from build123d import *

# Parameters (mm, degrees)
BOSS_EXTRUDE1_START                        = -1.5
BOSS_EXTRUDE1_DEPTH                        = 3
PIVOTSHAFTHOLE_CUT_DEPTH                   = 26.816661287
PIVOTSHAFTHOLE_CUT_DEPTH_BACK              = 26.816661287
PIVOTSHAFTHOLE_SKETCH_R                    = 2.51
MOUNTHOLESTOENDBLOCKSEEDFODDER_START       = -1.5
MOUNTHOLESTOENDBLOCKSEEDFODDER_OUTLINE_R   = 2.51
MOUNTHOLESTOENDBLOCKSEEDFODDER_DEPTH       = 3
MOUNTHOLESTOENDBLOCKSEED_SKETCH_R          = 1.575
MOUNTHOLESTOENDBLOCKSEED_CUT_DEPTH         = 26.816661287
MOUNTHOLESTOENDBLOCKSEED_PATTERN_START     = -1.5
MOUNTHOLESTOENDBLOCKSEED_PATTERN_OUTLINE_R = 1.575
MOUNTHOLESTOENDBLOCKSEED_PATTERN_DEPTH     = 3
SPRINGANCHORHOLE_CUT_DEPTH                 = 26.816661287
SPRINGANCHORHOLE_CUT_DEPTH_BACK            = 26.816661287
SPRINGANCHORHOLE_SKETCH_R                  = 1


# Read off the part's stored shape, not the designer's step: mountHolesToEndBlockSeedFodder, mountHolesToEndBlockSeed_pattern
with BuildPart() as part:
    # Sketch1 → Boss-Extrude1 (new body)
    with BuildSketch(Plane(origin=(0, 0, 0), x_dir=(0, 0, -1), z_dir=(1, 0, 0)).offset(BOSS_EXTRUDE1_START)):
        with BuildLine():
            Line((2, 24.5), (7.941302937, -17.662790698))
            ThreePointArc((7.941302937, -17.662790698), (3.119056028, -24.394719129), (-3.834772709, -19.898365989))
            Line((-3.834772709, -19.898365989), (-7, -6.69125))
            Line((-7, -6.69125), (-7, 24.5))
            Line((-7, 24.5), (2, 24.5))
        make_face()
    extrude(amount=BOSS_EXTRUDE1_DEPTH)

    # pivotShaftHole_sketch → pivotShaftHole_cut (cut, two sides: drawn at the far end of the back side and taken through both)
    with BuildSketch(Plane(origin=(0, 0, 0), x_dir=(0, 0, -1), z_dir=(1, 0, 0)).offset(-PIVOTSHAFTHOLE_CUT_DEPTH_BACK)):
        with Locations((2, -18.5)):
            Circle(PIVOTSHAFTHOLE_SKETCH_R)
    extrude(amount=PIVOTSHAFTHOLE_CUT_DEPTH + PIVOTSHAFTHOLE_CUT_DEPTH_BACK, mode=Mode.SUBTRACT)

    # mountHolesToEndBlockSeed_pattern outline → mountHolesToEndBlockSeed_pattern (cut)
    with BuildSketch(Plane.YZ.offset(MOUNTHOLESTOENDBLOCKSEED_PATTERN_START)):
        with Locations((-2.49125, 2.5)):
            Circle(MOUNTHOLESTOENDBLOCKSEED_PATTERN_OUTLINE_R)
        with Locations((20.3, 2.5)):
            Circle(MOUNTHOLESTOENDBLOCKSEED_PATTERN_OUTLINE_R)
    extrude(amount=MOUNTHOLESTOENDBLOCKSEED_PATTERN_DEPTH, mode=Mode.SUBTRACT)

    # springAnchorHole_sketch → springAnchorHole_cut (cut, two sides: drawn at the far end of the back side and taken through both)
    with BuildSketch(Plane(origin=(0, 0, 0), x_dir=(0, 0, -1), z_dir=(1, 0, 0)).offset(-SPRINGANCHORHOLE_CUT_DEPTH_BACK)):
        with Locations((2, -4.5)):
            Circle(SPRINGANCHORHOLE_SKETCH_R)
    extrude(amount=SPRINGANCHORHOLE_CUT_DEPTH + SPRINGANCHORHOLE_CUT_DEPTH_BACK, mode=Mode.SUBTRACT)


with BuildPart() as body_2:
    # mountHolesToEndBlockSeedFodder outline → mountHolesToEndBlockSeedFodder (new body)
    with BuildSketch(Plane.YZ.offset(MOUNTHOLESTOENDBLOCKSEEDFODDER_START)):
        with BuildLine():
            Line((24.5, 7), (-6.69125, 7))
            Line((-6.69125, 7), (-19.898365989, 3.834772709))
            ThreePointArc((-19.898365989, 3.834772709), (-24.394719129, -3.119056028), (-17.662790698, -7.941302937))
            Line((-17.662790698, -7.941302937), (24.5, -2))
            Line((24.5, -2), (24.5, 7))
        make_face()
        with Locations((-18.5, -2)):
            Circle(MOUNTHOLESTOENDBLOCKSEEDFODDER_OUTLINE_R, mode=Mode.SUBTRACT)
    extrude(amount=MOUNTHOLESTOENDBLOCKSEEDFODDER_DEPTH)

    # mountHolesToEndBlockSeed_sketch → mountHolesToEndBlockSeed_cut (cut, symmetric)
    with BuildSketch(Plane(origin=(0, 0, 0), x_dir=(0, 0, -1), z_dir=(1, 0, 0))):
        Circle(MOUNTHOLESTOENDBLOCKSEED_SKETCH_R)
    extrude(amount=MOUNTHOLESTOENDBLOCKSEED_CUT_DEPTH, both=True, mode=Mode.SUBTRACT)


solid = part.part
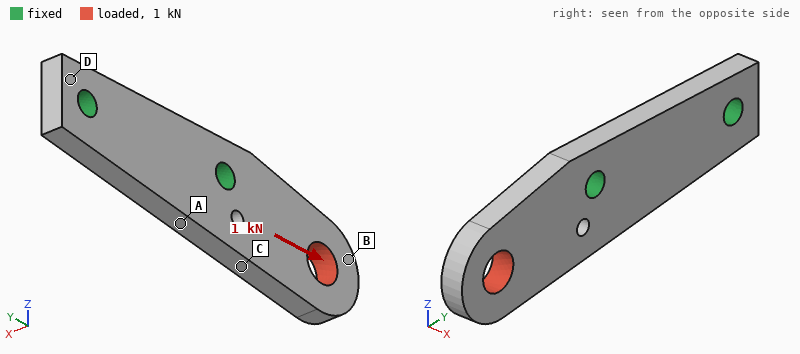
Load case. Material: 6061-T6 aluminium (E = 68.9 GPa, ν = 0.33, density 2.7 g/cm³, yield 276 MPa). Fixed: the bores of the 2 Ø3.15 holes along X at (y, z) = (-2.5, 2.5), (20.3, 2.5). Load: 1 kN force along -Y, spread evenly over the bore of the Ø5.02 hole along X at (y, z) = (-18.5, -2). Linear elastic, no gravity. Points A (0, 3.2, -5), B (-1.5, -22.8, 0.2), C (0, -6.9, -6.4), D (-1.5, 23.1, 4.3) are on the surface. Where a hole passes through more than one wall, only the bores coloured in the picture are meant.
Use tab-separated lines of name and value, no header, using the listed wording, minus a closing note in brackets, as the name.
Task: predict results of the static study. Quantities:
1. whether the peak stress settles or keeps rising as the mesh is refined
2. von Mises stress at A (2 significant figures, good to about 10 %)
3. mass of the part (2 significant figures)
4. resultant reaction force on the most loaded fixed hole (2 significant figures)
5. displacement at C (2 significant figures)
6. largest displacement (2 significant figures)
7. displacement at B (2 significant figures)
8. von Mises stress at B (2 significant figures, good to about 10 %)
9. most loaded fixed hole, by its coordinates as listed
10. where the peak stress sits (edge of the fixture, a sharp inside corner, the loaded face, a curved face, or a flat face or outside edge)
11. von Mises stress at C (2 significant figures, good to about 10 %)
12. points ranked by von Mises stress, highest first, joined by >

whether the peak stress settles or keeps rising as the mesh is refined	keeps rising
von Mises stress at A	39 MPa
mass of the part	4.2 g
resultant reaction force on the most loaded fixed hole	820 N
displacement at C	14 µm
largest displacement	35 µm
displacement at B	31 µm
von Mises stress at B	21 MPa
most loaded fixed hole, by its coordinates as listed	(-2.5, 2.5)
where the peak stress sits	edge of the fixture
von Mises stress at C	54 MPa
points ranked by von Mises stress, highest first, joined by >	C > A > B > D
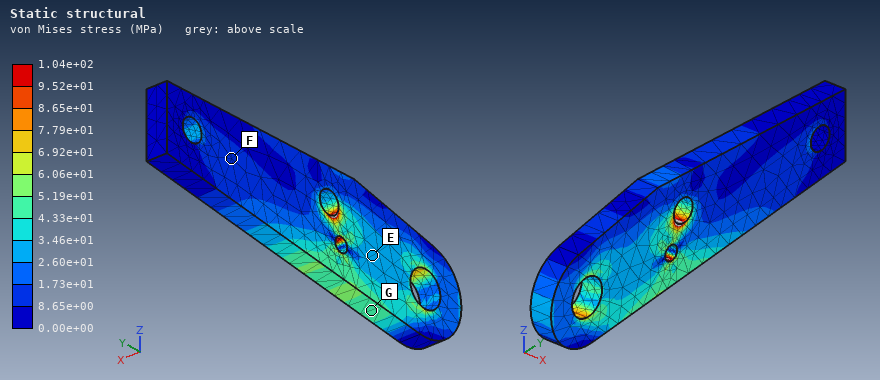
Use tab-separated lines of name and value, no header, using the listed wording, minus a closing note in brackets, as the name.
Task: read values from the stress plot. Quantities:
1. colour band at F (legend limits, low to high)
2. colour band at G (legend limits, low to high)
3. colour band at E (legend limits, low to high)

colour band at F	8.65e+00 to 1.73e+01 MPa
colour band at G	4.33e+01 to 5.19e+01 MPa
colour band at E	2.60e+01 to 3.46e+01 MPa
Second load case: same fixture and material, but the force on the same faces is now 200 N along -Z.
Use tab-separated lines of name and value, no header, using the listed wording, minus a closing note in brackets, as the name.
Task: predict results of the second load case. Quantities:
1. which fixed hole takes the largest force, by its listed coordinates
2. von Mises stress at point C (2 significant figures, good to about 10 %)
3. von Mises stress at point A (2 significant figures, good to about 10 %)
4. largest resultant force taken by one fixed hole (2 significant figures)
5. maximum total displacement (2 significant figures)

which fixed hole takes the largest force, by its listed coordinates	(-2.5, 2.5)
von Mises stress at point C	28 MPa
von Mises stress at point A	23 MPa
largest resultant force taken by one fixed hole	300 N
maximum total displacement	29 µm
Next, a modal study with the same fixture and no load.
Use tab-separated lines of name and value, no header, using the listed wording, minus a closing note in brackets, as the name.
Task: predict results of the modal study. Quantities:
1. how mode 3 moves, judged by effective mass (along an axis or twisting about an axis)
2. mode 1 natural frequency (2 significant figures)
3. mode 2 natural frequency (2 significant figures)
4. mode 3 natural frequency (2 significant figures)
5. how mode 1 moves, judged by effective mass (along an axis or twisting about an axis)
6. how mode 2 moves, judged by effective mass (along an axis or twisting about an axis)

how mode 3 moves, judged by effective mass	twisting about Y
mode 1 natural frequency	5900 Hz
mode 2 natural frequency	15 kHz
mode 3 natural frequency	17 kHz
how mode 1 moves, judged by effective mass	along X
how mode 2 moves, judged by effective mass	along Z
